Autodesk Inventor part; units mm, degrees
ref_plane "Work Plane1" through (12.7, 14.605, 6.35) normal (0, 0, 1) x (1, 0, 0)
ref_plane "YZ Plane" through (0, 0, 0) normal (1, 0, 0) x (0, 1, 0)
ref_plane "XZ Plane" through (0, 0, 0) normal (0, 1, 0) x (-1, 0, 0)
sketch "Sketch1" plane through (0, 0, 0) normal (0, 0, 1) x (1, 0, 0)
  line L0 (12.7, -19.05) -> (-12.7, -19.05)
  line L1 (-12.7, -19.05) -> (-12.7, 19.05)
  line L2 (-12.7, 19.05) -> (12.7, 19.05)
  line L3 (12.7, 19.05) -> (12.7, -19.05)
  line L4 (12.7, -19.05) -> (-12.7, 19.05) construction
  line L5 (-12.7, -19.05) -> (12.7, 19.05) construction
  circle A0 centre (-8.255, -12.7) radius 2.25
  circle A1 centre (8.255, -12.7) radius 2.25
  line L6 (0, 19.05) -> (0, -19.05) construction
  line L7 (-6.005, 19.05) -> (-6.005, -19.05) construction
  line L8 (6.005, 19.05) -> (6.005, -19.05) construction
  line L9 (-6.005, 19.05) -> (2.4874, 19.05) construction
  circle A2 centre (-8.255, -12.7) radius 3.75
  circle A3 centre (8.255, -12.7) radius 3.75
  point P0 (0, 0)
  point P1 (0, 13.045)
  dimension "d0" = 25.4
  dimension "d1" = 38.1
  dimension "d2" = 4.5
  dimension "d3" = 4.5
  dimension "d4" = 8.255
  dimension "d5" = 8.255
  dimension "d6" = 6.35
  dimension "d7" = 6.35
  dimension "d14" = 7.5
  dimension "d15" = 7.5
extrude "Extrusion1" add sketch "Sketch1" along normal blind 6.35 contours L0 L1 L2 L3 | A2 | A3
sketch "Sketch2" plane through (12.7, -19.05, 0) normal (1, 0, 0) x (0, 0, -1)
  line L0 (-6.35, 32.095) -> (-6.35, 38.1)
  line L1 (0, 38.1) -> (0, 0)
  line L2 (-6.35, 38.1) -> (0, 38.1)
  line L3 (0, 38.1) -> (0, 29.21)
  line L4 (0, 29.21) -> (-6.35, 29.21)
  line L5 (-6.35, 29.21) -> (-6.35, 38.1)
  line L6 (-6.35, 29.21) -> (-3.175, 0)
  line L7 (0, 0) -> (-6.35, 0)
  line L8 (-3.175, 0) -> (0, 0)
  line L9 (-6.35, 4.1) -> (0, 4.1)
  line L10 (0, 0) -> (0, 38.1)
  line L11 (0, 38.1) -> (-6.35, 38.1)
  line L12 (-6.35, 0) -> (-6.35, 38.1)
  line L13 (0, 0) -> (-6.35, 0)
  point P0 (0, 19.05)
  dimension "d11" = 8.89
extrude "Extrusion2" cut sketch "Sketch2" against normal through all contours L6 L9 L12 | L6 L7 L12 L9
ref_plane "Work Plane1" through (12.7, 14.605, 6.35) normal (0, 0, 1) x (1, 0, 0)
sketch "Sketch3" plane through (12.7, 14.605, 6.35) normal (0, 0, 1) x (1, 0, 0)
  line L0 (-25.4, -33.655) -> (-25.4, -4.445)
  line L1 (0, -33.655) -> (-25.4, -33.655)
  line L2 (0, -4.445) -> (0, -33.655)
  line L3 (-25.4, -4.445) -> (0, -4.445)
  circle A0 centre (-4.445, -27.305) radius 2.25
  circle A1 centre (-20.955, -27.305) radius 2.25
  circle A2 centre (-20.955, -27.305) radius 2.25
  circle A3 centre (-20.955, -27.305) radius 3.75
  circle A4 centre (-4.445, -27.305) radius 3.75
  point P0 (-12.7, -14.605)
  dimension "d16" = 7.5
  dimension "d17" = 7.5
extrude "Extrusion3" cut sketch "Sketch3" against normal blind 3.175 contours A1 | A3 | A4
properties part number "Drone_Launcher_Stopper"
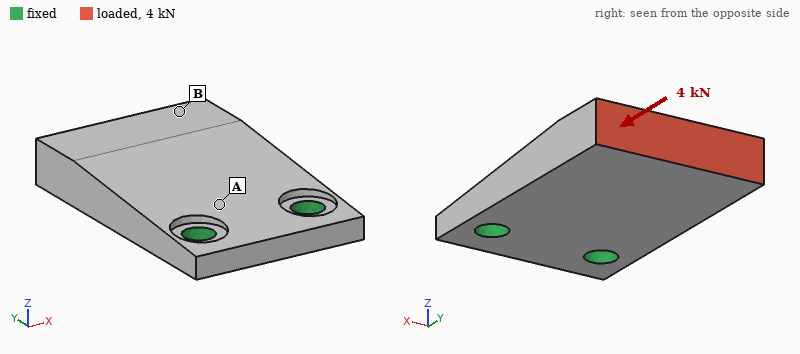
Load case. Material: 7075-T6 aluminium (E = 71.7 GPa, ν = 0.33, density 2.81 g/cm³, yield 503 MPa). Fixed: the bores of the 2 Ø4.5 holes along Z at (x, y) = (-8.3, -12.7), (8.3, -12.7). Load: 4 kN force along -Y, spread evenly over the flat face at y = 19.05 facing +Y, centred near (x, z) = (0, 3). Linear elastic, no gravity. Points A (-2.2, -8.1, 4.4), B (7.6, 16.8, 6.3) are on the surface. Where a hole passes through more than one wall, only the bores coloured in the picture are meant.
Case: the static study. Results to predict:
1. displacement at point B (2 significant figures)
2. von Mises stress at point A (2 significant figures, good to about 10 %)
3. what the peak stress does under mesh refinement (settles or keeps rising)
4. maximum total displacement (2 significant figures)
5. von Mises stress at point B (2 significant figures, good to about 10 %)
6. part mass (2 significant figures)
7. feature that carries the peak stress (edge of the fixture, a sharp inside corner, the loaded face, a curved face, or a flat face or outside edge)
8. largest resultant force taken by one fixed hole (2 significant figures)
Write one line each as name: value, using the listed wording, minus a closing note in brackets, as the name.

displacement at point B: 0.13 mm
von Mises stress at point A: 72 MPa
what the peak stress does under mesh refinement: keeps rising
maximum total displacement: 0.14 mm
von Mises stress at point B: 25 MPa
part mass: 14 g
feature that carries the peak stress: edge of the fixture
largest resultant force taken by one fixed hole: 2.0 kN
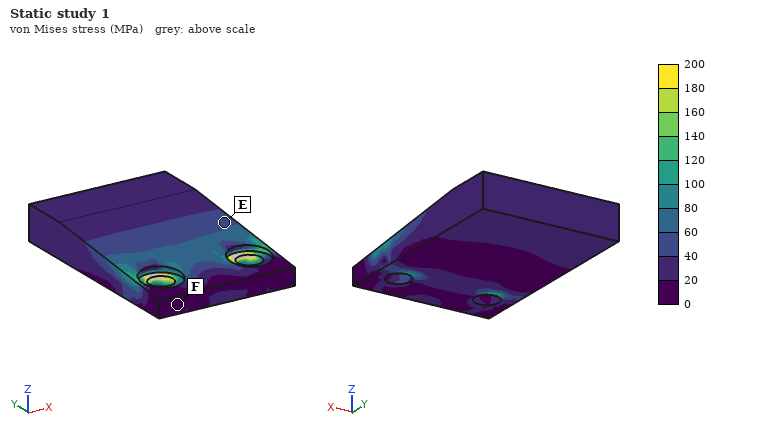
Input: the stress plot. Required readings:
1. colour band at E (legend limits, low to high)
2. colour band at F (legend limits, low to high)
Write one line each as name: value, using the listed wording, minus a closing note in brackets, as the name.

colour band at E: 40 to 60 MPa
colour band at F: 0 to 20 MPa
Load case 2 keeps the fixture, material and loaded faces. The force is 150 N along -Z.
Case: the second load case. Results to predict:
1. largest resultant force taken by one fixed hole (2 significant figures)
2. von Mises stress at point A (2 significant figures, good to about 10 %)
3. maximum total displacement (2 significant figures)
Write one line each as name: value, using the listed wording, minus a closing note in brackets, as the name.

largest resultant force taken by one fixed hole: 78 N
von Mises stress at point A: 45 MPa
maximum total displacement: 0.12 mm
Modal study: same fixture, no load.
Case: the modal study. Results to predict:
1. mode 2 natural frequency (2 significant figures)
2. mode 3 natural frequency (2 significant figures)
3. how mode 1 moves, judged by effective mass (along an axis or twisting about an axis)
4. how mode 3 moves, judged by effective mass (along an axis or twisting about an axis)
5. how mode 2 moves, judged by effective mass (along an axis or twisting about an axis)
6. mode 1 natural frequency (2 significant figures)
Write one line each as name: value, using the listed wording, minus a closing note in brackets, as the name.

mode 2 natural frequency: 9800 Hz
mode 3 natural frequency: 13 kHz
how mode 1 moves, judged by effective mass: along Z
how mode 3 moves, judged by effective mass: along X
how mode 2 moves, judged by effective mass: twisting about Y
mode 1 natural frequency: 2900 Hz
